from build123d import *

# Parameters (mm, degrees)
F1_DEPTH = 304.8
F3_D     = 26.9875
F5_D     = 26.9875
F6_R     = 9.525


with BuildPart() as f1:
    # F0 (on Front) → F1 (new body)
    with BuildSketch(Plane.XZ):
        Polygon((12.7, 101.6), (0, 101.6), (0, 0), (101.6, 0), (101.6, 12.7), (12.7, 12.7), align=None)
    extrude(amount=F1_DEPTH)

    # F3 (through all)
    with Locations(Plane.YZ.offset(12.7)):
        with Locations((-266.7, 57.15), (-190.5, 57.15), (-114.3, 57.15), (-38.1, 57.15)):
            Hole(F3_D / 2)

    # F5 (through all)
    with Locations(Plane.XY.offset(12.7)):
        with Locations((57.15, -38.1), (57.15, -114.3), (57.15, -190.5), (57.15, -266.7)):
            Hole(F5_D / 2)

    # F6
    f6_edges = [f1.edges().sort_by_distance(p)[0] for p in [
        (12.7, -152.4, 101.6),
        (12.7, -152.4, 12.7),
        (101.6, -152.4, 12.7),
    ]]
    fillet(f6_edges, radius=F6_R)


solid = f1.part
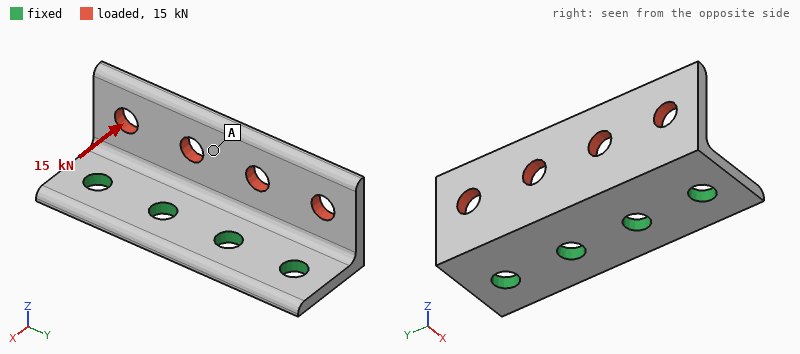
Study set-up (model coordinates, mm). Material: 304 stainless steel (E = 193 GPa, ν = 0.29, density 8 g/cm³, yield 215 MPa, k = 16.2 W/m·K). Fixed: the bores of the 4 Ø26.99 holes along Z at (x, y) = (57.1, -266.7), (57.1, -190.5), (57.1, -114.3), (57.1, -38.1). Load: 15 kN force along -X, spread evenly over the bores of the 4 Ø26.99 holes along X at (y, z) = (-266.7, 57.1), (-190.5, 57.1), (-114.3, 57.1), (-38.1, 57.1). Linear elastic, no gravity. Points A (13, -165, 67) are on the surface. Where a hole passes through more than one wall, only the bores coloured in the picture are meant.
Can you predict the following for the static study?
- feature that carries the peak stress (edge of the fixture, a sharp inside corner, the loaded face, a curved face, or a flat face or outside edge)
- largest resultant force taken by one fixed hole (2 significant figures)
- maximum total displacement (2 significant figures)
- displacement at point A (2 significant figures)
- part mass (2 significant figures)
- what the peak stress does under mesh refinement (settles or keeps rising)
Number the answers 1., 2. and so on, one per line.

1. edge of the fixture
2. 3.9 kN
3. 0.37 mm
4. 0.22 mm
5. 5.4 kg
6. keeps rising
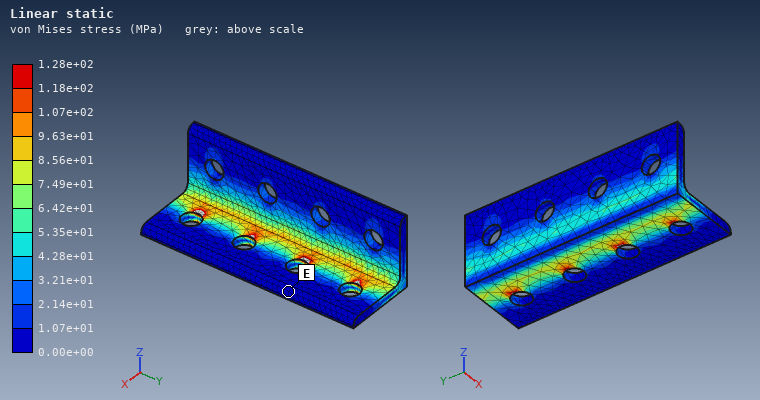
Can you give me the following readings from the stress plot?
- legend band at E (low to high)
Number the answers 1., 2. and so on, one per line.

1. 0.00e+00 to 1.07e+01 MPa
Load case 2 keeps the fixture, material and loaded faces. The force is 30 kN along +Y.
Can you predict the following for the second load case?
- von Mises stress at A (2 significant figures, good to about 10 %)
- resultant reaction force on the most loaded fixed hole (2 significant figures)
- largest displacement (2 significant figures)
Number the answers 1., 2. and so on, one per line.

1. 21 MPa
2. 10 kN
3. 0.13 mm
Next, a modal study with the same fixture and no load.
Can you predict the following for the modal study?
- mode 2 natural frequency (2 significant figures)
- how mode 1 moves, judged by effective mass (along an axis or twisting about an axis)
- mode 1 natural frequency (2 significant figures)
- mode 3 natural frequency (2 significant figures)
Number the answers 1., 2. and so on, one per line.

1. 1000 Hz
2. along X
3. 740 Hz
4. 1900 Hz
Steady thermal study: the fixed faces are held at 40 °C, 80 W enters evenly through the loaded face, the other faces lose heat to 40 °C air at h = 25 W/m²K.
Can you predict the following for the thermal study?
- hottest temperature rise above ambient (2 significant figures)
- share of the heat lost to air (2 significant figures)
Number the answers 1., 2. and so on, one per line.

1. 53 K
2. 70 %
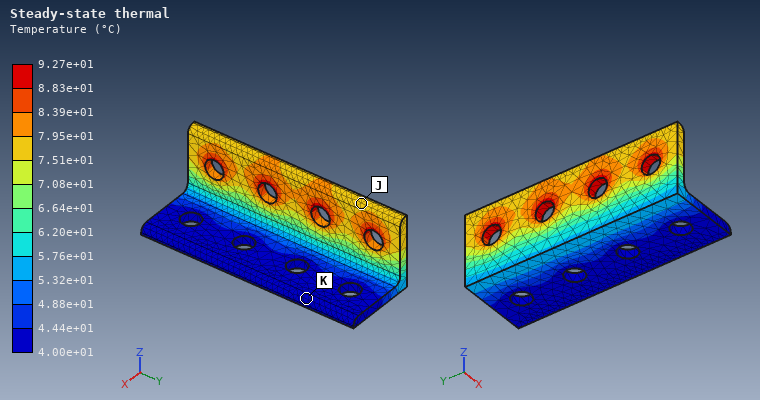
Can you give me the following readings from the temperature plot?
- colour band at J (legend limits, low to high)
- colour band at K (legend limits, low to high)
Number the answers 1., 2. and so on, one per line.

1. 7.51e+01 to 7.95e+01 °C
2. 4.00e+01 to 4.44e+01 °C
